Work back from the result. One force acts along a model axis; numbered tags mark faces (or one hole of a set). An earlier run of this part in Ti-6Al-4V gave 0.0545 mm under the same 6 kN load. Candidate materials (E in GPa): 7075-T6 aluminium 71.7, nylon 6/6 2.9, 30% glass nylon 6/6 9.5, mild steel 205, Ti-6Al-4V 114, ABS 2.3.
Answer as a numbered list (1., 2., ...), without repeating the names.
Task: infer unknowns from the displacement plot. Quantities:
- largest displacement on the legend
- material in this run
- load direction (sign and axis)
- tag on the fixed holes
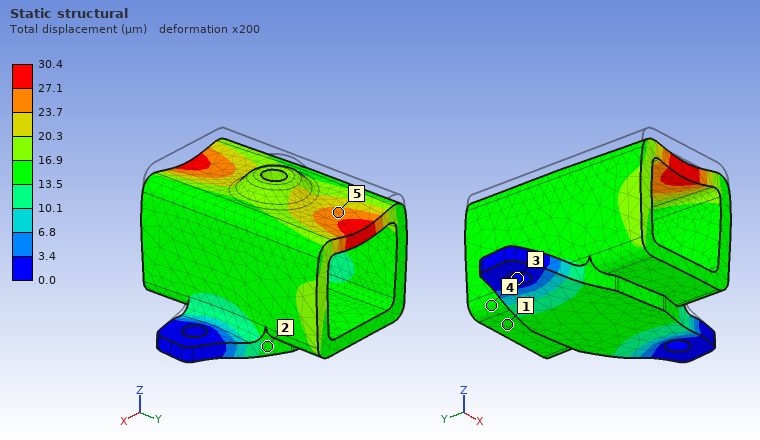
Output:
1. 30.4 µm
2. mild steel
3. -Z
4. 3
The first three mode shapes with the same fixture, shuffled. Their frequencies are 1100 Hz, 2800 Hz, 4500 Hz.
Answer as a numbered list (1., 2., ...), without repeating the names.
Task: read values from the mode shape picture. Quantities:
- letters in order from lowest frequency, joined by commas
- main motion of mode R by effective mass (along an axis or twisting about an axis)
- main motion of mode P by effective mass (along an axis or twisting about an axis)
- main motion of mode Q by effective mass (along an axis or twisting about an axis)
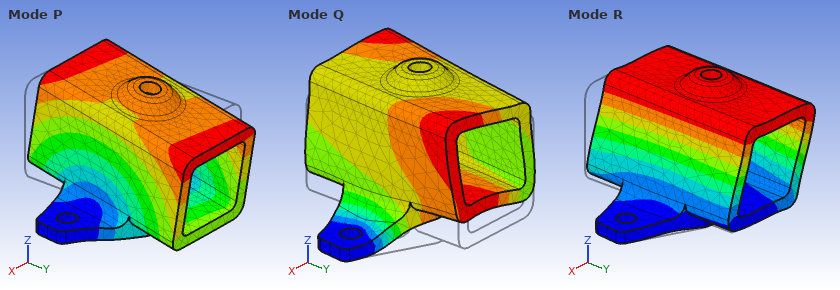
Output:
1. P, R, Q
2. along X
3. along Y
4. along Z
